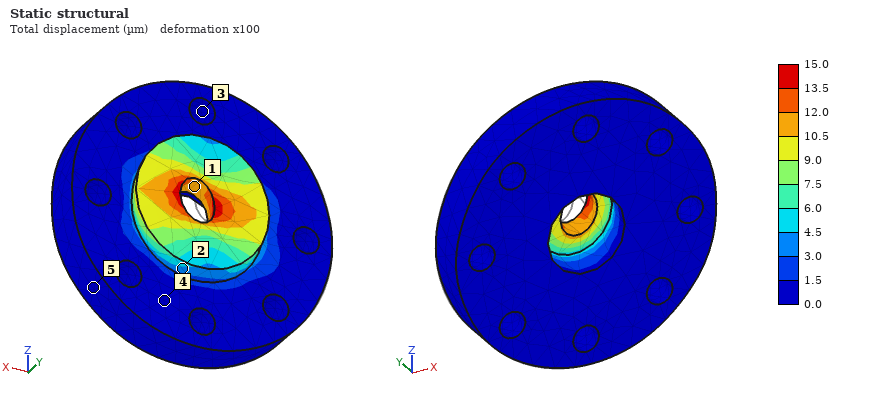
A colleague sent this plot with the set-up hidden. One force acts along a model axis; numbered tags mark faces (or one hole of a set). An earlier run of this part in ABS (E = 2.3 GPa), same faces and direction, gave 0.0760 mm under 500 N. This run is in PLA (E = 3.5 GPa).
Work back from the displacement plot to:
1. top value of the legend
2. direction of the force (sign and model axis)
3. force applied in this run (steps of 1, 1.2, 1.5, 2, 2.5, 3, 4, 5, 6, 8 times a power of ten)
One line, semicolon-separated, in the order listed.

15.0 µm; +X; 150 N
